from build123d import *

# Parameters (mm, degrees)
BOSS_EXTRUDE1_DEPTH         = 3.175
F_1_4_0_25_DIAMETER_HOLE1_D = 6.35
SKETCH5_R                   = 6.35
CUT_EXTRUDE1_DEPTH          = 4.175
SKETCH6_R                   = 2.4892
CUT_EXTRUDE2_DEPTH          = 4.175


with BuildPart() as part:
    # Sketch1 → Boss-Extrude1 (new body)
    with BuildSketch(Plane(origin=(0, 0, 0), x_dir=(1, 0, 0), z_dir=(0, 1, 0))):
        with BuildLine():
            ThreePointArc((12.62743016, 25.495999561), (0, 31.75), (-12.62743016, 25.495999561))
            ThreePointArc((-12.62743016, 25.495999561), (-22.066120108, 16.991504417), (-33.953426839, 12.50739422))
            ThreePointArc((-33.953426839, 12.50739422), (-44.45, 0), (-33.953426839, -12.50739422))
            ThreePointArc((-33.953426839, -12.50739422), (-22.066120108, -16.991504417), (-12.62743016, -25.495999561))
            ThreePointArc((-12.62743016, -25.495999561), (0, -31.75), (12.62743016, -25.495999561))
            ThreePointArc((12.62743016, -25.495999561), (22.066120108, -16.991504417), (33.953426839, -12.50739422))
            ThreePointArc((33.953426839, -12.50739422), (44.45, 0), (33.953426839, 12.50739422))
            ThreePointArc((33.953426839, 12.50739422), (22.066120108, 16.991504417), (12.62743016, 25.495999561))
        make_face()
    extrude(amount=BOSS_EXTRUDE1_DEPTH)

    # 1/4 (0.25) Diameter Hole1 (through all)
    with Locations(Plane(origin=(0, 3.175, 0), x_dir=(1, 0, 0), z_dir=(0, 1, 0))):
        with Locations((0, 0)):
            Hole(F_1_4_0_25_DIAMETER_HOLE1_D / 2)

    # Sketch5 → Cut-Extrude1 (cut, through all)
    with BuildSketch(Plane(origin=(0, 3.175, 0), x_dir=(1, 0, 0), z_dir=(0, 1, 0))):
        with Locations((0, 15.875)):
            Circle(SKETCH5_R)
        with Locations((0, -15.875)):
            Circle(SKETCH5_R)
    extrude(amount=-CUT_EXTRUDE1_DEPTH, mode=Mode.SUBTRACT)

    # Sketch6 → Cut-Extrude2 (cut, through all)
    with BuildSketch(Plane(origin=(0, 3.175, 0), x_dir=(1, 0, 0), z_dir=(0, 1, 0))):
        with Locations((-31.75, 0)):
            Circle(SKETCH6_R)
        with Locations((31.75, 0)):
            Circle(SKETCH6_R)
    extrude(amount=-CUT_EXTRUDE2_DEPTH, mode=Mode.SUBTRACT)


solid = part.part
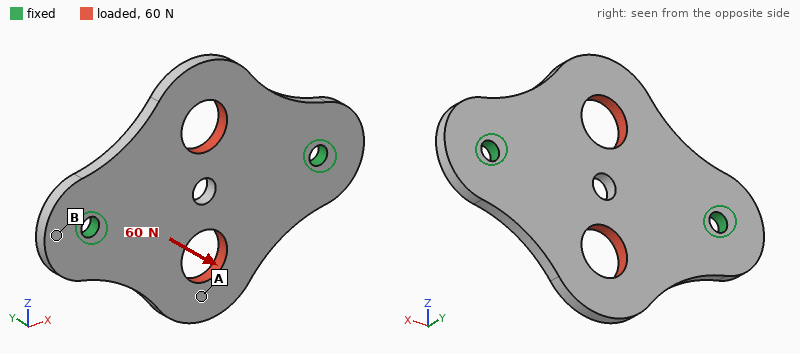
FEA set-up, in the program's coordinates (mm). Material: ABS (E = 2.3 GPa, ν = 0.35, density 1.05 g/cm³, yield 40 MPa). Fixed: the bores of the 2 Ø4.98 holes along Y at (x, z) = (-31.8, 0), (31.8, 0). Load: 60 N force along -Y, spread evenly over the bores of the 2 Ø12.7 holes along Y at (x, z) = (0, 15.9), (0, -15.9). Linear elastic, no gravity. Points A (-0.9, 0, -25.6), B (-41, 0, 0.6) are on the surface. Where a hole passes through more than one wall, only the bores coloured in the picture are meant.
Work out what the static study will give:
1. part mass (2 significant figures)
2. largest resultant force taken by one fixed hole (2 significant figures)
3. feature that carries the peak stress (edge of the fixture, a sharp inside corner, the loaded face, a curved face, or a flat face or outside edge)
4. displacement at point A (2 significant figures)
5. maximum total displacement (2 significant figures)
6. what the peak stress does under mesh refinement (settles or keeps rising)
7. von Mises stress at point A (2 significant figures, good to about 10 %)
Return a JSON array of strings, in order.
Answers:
["10 g", "30 N", "edge of the fixture", "0.60 mm", "0.67 mm", "keeps rising", "6.0 MPa"]
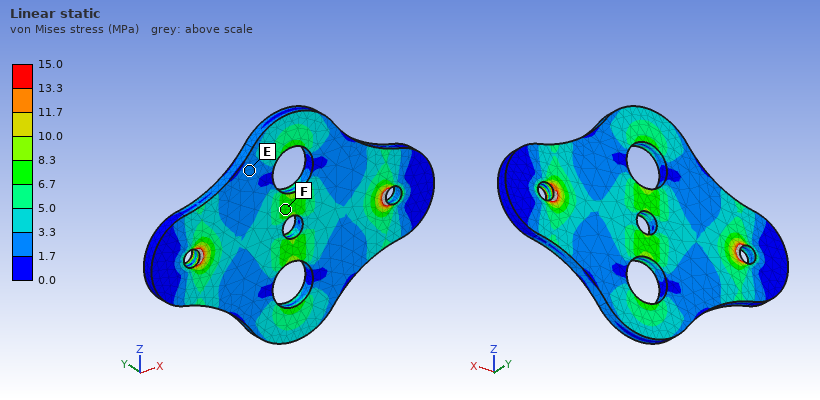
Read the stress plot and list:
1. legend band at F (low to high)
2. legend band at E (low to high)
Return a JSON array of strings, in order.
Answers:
["6.7 to 8.3 MPa", "1.7 to 3.3 MPa"]
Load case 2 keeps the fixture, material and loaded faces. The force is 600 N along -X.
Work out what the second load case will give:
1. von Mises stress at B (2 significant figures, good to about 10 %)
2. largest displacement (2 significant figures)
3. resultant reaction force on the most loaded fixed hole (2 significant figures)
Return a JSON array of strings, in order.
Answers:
["1.9 MPa", "74 µm", "300 N"]
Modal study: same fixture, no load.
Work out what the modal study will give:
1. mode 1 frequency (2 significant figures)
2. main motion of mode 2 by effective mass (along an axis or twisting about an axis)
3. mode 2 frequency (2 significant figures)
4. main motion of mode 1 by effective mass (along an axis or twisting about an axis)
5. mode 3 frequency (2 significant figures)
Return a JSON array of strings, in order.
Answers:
["680 Hz", "along Y", "810 Hz", "twisting about X", "1900 Hz"]
